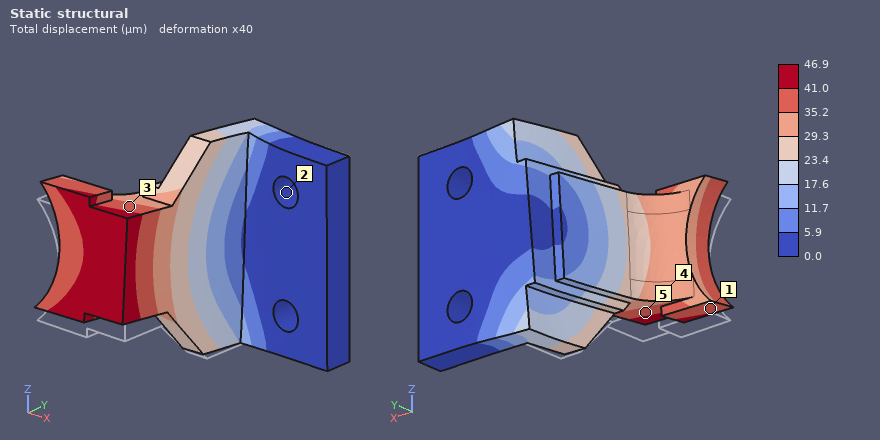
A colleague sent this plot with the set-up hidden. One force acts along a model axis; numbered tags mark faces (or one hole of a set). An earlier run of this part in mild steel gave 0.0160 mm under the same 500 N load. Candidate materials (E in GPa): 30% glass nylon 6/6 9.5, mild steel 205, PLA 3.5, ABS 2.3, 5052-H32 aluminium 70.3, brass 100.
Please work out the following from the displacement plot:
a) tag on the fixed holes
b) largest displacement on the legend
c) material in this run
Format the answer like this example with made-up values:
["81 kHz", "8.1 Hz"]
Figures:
["2", "46.9 µm", "5052-H32 aluminium"]
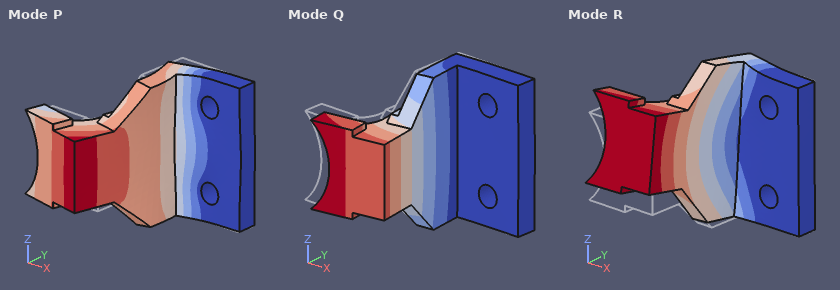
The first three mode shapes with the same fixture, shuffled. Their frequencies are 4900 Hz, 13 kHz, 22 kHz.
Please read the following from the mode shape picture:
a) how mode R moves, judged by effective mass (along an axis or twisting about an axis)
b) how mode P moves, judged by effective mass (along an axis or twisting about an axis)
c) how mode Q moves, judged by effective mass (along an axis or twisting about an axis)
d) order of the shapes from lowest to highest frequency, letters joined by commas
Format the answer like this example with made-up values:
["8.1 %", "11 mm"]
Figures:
["along Z", "along Y", "along X", "Q, R, P"]
